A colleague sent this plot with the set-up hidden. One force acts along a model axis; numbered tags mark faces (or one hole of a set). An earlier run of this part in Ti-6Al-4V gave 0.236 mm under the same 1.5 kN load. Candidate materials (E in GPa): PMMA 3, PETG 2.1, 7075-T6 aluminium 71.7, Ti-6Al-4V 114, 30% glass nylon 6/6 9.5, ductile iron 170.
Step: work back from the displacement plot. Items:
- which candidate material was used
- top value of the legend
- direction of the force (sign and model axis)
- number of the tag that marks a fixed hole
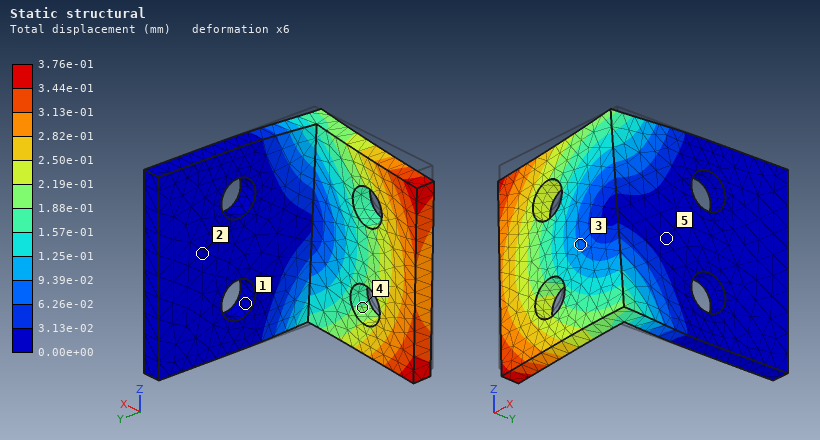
7075-T6 aluminium
3.76e-01 mm
-Z
1
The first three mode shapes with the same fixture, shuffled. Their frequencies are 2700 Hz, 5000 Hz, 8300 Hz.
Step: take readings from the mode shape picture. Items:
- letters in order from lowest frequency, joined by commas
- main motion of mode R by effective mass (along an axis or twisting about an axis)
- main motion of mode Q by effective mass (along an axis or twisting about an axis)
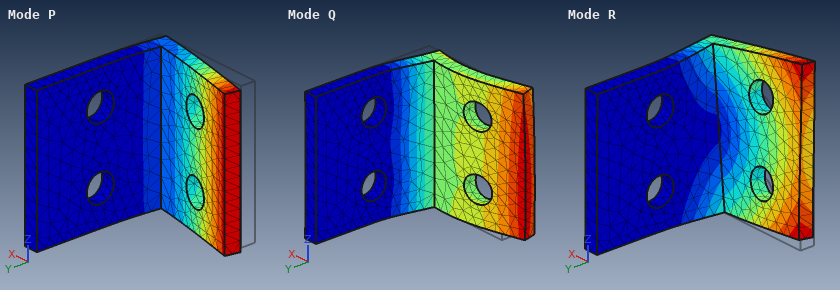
P, R, Q
along Z
along X
